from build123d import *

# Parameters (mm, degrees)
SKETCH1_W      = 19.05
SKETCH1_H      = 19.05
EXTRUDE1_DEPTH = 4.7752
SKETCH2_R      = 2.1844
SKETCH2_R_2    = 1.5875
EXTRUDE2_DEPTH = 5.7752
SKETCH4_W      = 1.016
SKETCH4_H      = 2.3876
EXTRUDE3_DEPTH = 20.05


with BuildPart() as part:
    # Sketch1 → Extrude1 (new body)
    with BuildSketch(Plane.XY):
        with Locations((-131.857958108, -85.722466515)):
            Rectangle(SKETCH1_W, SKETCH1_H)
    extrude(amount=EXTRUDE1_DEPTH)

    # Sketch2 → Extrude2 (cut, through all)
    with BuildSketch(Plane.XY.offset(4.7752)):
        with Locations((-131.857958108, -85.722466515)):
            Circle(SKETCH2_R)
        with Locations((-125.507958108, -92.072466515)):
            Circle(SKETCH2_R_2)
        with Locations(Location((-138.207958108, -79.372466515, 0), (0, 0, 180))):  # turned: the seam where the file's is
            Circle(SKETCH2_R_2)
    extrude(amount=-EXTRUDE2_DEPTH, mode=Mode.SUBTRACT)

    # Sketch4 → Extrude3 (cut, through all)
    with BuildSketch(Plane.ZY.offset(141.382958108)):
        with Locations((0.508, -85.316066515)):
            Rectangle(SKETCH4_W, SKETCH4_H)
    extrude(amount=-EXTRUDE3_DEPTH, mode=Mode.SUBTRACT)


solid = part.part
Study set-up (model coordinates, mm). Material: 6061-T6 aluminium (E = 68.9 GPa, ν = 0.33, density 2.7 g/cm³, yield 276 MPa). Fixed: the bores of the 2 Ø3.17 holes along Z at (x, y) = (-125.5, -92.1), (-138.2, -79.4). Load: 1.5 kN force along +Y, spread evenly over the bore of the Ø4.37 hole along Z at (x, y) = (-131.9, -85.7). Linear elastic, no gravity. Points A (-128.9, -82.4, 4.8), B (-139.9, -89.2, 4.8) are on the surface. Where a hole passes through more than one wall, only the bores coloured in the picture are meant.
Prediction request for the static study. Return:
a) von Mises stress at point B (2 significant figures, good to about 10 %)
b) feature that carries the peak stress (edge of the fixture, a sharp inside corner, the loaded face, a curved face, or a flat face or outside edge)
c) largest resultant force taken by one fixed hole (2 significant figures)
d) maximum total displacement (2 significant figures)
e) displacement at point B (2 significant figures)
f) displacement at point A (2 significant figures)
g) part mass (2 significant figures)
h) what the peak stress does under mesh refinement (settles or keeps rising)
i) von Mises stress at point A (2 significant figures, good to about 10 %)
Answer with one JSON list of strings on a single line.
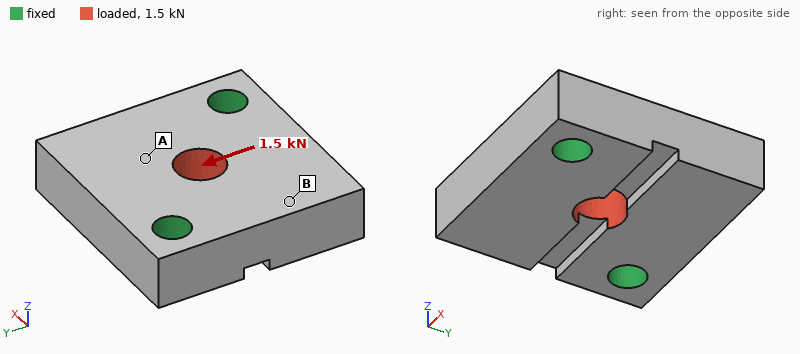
["8.4 MPa", "edge of the fixture", "760 N", "3.9 µm", "1.8 µm", "3.0 µm", "4.2 g", "keeps rising", "17 MPa"]
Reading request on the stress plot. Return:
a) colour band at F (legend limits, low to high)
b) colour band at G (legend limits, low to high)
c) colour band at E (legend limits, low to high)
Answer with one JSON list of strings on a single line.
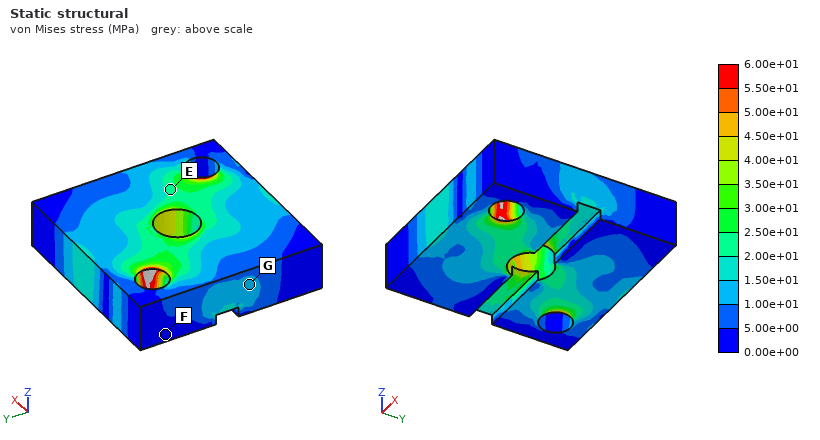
["0.00e+00 to 5.00e+00 MPa", "1.00e+01 to 1.50e+01 MPa", "2.00e+01 to 2.50e+01 MPa"]
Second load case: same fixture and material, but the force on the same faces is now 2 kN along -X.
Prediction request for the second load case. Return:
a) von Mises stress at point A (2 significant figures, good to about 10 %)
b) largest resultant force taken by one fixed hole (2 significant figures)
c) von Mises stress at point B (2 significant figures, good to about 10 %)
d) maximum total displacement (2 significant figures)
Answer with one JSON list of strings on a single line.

["22 MPa", "1.0 kN", "15 MPa", "5.1 µm"]
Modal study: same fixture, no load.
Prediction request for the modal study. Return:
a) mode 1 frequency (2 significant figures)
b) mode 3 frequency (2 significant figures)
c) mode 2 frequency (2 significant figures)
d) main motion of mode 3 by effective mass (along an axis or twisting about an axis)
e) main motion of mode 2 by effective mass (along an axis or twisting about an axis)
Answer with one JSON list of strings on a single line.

["24 kHz", "66 kHz", "29 kHz", "along Y", "along Z"]
